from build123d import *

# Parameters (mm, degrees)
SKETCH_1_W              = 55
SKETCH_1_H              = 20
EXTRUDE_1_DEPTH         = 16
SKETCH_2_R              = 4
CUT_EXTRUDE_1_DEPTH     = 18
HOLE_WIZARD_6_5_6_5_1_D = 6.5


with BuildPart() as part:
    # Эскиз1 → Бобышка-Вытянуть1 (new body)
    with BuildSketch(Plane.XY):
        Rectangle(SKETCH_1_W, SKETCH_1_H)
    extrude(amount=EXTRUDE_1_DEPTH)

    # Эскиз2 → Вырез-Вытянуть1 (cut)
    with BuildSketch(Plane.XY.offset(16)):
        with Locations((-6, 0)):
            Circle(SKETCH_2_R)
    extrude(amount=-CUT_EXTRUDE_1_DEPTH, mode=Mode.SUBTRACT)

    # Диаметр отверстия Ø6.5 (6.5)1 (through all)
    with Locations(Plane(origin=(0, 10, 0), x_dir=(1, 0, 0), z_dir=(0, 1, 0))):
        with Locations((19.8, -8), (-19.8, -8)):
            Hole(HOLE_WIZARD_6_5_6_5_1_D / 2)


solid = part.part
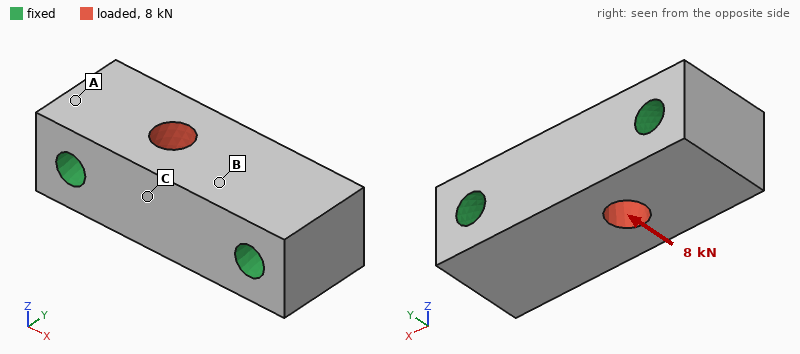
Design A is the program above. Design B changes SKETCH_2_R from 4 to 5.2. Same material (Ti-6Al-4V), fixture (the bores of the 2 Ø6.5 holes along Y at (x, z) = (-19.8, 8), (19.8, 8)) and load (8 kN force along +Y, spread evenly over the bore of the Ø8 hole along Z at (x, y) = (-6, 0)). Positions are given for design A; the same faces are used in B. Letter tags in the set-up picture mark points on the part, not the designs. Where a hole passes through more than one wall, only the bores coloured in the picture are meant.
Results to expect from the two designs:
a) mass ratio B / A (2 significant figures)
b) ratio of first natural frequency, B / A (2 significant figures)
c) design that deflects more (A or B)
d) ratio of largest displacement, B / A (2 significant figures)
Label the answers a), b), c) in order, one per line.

a) 0.96
b) 1.00
c) B
d) 1.1
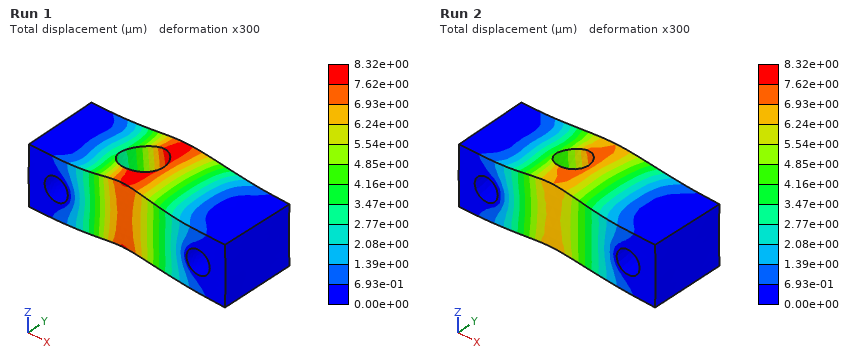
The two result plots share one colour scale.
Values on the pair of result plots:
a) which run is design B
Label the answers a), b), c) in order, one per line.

a) Run 1
